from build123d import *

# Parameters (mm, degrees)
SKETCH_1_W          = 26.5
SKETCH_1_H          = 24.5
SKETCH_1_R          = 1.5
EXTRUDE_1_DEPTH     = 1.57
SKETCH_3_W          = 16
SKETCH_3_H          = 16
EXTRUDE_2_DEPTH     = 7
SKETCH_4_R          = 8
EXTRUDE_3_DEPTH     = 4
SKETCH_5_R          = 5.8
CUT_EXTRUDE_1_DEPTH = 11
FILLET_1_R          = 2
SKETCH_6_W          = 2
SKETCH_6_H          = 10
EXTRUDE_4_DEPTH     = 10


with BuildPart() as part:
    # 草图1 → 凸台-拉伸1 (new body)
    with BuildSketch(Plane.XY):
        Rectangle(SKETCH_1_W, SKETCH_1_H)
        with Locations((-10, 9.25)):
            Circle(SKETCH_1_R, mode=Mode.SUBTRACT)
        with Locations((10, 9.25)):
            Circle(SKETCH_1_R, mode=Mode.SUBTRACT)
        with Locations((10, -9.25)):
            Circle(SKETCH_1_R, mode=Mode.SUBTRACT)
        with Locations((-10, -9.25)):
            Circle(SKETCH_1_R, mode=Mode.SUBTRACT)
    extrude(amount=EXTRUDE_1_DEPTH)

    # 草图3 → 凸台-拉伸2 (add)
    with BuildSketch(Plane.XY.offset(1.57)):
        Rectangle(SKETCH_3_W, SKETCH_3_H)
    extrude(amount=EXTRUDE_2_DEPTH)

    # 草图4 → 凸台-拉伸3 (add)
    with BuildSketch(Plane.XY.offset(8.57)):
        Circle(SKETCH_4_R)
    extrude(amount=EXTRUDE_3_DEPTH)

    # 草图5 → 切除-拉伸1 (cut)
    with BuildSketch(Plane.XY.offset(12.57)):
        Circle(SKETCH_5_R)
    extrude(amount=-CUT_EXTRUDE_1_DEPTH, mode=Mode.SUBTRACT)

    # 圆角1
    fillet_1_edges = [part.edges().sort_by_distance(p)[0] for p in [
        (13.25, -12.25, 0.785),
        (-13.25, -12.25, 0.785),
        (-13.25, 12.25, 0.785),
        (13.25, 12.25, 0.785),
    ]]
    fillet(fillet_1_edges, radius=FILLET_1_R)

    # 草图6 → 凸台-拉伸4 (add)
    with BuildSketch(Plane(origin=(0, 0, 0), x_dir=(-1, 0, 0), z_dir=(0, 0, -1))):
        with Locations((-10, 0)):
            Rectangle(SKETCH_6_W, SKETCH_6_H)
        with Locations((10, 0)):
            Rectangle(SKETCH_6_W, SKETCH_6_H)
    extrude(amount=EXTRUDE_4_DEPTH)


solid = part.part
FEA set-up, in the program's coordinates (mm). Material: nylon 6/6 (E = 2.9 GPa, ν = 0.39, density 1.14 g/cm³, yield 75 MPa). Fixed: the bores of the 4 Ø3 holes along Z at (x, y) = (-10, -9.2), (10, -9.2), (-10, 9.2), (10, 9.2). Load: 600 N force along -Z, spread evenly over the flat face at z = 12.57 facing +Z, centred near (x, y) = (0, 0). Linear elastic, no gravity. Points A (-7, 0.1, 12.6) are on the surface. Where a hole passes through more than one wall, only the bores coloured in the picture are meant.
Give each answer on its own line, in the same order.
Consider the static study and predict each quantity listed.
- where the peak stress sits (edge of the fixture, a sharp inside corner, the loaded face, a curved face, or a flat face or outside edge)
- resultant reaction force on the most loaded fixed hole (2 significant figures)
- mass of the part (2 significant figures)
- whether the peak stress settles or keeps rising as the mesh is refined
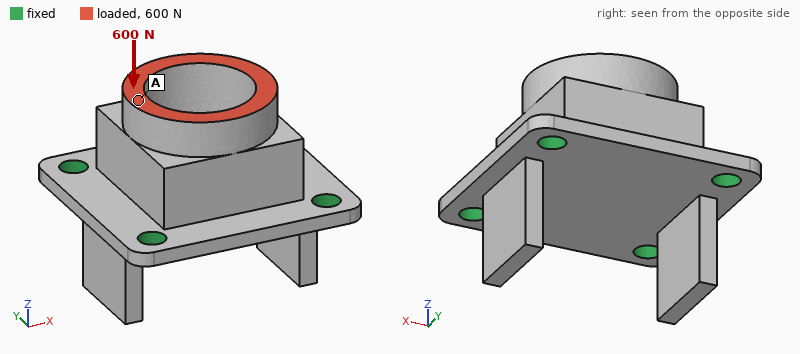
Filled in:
edge of the fixture
160 N
3.2 g
keeps rising
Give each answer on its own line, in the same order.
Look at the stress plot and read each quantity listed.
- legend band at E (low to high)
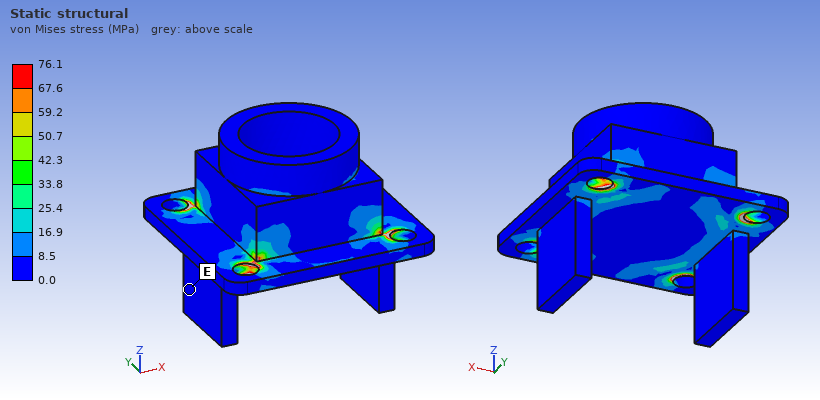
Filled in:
0.0 to 8.5 MPa
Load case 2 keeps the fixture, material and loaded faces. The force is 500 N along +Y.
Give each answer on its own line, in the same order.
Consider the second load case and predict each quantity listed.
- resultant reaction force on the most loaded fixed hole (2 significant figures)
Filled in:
240 N
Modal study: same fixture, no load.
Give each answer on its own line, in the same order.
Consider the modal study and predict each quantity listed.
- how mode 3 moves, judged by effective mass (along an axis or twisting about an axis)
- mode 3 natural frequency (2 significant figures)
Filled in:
along Z
7300 Hz
